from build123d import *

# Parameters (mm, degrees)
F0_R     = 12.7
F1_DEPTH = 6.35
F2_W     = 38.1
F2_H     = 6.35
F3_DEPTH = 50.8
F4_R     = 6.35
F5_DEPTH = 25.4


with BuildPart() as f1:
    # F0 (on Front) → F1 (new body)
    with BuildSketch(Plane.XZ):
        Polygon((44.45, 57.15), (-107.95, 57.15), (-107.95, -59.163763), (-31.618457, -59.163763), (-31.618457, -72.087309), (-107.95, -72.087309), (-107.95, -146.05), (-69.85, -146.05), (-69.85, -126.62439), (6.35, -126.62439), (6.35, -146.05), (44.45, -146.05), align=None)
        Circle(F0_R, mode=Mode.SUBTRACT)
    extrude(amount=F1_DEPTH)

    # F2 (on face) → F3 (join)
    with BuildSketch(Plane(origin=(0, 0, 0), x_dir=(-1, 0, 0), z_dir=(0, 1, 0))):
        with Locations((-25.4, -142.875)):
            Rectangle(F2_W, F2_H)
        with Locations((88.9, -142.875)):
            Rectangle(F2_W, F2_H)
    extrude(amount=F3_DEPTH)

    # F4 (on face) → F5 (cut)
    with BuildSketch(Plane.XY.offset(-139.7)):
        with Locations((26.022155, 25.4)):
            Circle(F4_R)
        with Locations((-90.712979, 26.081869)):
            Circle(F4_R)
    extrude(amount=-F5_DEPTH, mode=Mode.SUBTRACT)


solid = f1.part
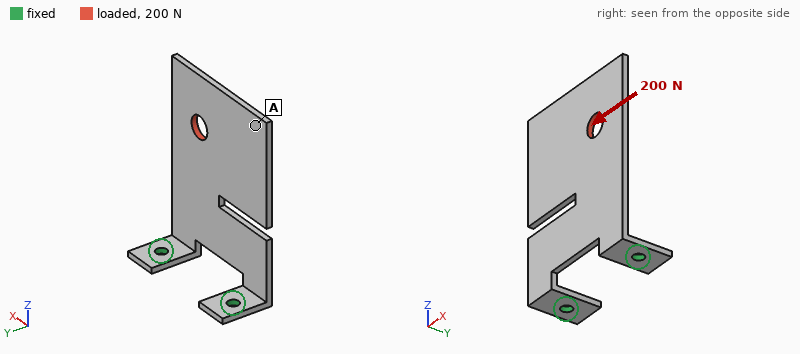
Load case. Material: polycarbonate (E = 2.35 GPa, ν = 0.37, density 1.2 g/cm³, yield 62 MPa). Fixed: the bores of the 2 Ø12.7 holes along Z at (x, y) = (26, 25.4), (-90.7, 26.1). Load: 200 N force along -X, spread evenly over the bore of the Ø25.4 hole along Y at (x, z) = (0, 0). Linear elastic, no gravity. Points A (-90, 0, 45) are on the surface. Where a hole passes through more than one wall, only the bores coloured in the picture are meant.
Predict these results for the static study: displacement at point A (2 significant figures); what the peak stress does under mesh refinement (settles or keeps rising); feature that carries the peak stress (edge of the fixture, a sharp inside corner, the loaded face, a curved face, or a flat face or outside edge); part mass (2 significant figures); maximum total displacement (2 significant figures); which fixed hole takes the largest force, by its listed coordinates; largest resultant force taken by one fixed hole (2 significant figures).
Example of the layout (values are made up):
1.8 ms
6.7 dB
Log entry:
2.2 mm
keeps rising
edge of the fixture
240 g
2.8 mm
(-90.7, 26.1)
270 N
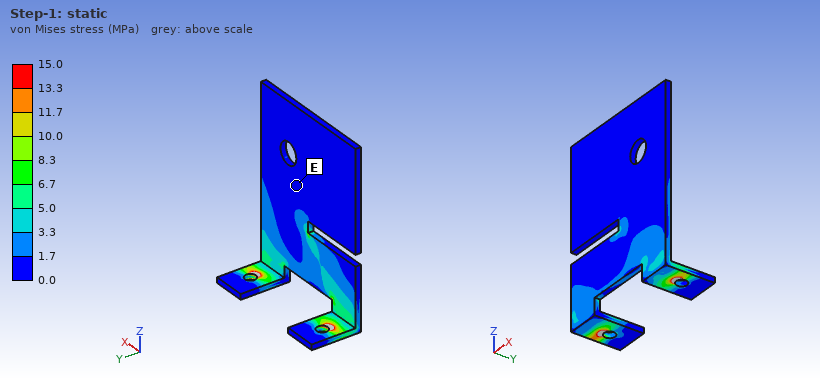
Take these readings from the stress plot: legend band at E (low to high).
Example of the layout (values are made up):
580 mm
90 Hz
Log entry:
0.0 to 1.7 MPa
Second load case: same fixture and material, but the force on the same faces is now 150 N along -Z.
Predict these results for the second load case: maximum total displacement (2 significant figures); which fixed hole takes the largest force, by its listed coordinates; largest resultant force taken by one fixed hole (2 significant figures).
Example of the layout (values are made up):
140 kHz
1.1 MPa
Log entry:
2.7 mm
(26, 25.4)
110 N
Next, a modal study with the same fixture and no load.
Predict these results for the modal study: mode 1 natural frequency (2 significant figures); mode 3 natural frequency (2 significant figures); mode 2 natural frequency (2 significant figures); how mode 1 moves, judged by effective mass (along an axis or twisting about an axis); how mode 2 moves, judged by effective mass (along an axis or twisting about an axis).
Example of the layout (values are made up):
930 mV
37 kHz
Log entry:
22 Hz
140 Hz
71 Hz
along Y
twisting about Z
